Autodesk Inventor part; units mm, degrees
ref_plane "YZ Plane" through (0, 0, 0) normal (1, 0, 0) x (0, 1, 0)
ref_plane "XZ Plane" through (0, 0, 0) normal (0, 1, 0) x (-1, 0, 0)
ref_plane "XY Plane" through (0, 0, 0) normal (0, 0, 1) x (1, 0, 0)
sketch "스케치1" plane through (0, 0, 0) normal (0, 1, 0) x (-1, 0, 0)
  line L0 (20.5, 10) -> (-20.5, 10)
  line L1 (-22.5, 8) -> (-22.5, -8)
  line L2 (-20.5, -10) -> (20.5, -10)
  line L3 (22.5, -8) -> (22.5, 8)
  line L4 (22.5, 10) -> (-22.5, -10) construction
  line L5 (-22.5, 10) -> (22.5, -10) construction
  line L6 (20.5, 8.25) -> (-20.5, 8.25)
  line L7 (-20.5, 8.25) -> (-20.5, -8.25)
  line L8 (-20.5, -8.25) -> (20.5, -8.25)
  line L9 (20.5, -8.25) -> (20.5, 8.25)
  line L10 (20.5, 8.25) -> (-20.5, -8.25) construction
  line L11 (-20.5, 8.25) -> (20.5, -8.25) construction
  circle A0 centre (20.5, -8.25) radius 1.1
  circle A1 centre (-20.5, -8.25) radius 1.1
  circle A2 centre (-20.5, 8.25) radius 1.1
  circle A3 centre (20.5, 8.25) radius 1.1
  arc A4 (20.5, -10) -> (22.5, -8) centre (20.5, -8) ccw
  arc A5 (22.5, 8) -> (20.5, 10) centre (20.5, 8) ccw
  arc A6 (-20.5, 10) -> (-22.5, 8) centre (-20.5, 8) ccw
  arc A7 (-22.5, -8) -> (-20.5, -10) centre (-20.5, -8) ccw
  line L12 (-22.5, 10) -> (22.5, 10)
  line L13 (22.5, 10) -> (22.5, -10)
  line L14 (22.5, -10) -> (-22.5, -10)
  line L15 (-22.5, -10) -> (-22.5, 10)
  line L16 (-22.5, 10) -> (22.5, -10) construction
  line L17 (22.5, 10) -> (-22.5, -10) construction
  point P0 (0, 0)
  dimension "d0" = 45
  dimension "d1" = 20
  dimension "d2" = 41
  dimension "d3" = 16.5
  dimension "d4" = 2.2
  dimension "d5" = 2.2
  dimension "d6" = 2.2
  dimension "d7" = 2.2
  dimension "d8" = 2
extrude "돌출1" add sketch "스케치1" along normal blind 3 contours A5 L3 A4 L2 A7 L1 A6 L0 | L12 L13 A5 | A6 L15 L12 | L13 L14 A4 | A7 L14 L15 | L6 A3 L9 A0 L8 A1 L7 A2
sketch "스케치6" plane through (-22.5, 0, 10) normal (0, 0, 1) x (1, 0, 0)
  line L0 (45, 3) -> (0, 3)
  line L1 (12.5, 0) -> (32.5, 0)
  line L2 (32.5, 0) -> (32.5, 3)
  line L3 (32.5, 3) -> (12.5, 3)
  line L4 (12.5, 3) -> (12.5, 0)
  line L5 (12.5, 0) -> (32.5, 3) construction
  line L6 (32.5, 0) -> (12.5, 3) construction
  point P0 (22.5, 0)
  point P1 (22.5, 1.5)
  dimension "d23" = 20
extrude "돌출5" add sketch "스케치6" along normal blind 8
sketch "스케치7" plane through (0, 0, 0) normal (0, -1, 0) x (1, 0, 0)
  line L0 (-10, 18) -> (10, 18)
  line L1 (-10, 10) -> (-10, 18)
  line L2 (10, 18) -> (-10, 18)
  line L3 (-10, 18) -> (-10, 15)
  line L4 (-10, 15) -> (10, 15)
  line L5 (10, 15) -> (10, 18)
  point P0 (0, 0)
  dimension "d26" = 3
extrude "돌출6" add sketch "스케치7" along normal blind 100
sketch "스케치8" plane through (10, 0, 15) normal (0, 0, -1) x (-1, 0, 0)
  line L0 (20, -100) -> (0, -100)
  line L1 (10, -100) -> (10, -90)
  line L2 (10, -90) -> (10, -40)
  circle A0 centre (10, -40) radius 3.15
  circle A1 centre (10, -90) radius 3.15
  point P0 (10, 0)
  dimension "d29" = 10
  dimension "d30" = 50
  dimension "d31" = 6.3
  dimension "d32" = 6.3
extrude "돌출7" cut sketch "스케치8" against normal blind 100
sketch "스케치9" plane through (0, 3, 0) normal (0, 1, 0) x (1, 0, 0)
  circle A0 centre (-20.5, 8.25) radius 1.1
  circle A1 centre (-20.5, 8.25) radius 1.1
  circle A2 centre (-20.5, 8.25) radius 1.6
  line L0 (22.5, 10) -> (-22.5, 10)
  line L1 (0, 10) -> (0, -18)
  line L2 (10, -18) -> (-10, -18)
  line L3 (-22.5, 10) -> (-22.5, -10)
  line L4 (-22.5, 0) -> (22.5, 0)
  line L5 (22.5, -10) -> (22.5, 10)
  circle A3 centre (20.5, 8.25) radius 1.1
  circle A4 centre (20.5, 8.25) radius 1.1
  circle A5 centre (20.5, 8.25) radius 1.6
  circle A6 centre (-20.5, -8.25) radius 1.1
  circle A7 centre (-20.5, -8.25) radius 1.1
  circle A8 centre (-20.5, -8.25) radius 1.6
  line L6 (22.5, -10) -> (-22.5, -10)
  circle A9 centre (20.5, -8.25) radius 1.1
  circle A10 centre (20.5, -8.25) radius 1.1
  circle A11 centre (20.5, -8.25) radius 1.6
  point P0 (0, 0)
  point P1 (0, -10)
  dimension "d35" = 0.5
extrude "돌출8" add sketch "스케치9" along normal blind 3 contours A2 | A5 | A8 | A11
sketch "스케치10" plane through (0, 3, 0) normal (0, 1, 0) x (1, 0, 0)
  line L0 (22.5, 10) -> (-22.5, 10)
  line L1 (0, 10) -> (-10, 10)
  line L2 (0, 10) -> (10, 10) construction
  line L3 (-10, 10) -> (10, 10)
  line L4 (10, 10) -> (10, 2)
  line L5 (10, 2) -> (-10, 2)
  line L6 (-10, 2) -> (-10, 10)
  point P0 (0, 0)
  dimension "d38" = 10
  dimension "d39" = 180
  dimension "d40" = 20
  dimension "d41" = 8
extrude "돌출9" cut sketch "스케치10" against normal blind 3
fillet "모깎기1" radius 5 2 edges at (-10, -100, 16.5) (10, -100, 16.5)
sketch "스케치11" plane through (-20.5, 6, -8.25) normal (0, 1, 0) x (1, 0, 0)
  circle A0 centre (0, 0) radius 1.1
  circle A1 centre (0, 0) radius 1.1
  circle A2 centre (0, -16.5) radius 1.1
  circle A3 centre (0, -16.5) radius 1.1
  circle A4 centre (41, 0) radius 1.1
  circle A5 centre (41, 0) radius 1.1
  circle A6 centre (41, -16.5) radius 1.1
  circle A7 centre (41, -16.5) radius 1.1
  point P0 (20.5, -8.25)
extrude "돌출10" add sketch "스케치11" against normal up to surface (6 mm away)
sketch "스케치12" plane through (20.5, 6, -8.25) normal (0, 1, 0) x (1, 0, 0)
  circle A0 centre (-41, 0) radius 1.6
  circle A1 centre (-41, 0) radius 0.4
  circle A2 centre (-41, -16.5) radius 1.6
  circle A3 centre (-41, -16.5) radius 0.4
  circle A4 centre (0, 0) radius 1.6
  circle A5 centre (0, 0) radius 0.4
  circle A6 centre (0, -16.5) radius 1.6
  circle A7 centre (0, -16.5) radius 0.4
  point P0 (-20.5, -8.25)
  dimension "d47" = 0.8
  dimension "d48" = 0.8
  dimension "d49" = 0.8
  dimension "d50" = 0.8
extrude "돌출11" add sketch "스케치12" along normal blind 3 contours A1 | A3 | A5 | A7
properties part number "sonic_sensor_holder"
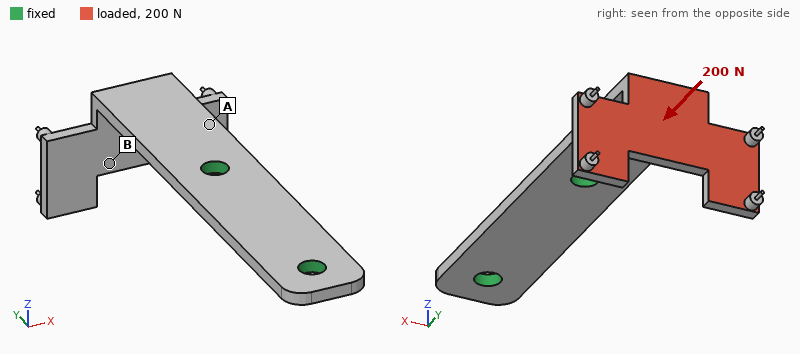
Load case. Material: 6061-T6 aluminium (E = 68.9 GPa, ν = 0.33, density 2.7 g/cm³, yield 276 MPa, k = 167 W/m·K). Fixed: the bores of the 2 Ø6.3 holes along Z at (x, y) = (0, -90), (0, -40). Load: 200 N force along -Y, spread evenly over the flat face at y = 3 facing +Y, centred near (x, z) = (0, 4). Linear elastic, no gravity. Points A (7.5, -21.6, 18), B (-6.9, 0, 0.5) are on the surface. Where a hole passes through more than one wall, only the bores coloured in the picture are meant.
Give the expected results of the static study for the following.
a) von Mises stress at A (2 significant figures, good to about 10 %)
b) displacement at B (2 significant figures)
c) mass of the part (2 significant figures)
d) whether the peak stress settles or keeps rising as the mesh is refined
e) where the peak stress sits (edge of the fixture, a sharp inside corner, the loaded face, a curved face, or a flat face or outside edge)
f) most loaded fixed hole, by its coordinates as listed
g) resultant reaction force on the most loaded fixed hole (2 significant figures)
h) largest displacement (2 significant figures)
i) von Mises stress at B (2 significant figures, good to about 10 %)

82 MPa
0.81 mm
23 g
keeps rising
edge of the fixture
(0, -40)
190 N
1.3 mm
20 MPa
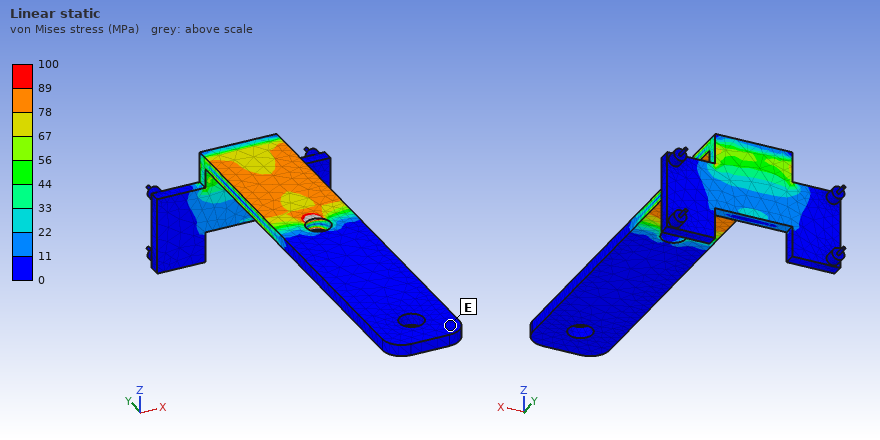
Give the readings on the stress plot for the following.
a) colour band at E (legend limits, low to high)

0 to 11 MPa
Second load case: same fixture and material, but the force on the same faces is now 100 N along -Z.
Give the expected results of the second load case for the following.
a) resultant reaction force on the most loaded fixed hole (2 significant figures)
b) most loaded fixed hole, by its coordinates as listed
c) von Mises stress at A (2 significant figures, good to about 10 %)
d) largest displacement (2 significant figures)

100 N
(0, -40)
82 MPa
1.1 mm
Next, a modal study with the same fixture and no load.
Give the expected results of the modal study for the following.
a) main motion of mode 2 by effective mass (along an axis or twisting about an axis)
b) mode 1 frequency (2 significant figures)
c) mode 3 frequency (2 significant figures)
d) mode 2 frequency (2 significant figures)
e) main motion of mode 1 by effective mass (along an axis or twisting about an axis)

along X
580 Hz
1900 Hz
970 Hz
along Z
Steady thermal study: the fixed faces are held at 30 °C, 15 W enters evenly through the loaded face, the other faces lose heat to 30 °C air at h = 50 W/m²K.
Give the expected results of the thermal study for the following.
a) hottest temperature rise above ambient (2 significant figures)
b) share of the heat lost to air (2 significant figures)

53 K
37 %
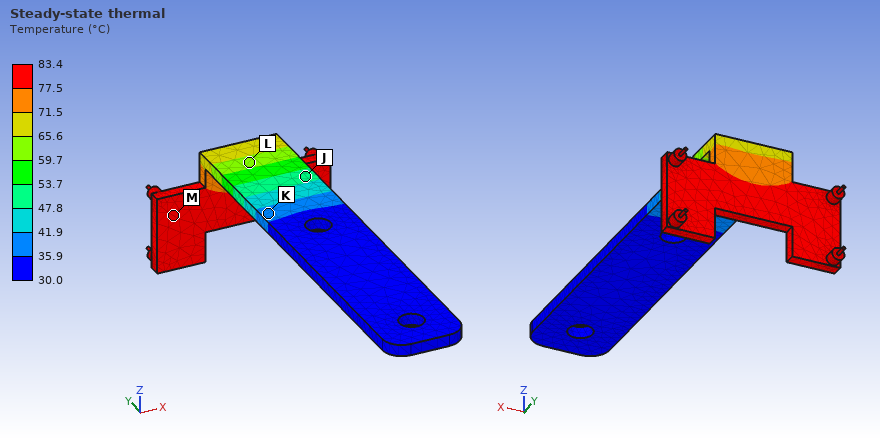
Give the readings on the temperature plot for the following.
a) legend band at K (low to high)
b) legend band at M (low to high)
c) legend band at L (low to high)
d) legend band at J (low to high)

35.9 to 41.9 °C
77.5 to 83.4 °C
59.7 to 65.6 °C
47.8 to 53.7 °C
